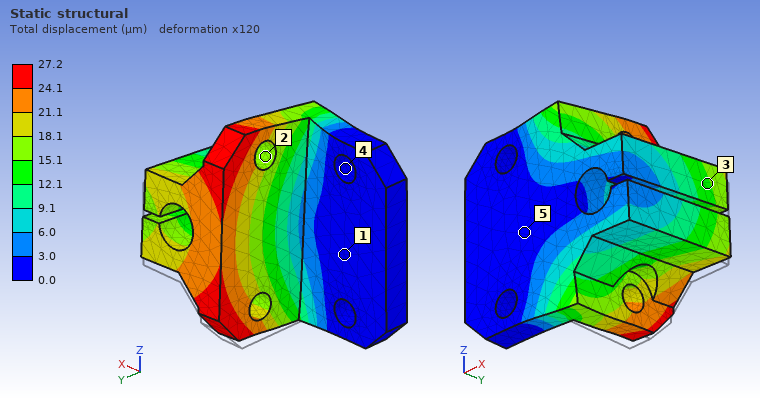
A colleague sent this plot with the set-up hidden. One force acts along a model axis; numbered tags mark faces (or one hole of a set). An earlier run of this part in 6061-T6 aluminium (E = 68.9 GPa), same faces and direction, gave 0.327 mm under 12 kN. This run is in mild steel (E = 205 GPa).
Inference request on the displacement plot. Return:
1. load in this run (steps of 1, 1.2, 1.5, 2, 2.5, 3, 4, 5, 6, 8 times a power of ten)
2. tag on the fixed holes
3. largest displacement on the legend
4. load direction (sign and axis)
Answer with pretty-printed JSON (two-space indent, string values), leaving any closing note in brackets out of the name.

{
  "load in this run": "3 kN",
  "tag on the fixed holes": "4",
  "largest displacement on the legend": "27.2 µm",
  "load direction": "+Z"
}
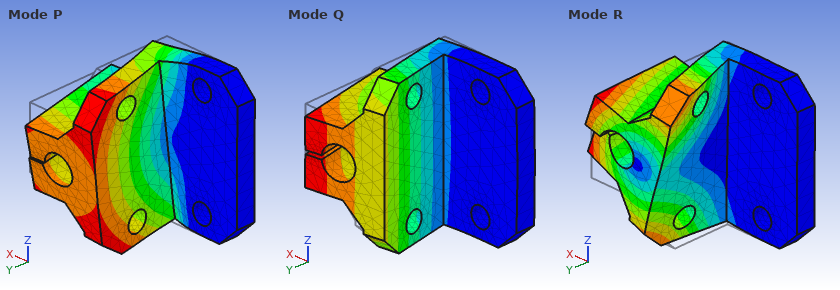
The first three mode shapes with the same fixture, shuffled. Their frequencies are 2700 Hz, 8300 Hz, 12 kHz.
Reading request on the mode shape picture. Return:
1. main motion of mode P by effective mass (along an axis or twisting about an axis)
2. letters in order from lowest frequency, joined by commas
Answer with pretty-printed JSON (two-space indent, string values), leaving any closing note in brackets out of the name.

{
  "main motion of mode P by effective mass": "along Z",
  "letters in order from lowest frequency, joined by commas": "Q, P, R"
}
